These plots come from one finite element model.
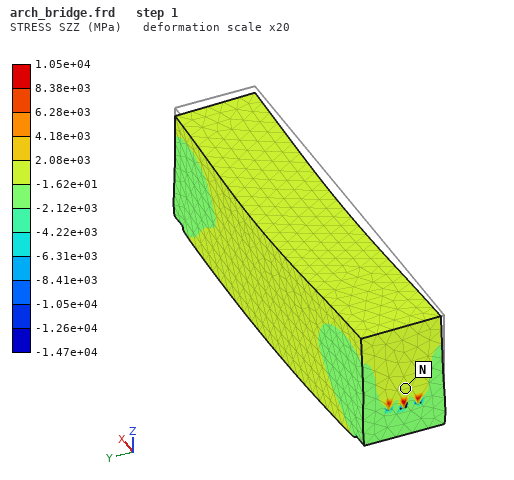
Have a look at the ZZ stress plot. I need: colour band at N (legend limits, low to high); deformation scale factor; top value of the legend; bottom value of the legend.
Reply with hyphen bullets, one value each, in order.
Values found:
- -1.62e+01 to 2.08e+03 MPa
- 20
- 1.05e+04 MPa
- -1.47e+04 MPa
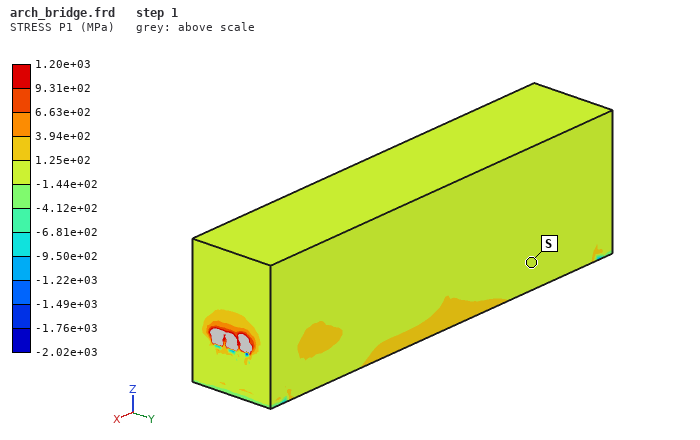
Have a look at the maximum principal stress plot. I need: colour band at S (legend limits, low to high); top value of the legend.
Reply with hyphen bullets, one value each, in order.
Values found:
- -1.44e+02 to 1.25e+02 MPa
- 1.20e+03 MPa
